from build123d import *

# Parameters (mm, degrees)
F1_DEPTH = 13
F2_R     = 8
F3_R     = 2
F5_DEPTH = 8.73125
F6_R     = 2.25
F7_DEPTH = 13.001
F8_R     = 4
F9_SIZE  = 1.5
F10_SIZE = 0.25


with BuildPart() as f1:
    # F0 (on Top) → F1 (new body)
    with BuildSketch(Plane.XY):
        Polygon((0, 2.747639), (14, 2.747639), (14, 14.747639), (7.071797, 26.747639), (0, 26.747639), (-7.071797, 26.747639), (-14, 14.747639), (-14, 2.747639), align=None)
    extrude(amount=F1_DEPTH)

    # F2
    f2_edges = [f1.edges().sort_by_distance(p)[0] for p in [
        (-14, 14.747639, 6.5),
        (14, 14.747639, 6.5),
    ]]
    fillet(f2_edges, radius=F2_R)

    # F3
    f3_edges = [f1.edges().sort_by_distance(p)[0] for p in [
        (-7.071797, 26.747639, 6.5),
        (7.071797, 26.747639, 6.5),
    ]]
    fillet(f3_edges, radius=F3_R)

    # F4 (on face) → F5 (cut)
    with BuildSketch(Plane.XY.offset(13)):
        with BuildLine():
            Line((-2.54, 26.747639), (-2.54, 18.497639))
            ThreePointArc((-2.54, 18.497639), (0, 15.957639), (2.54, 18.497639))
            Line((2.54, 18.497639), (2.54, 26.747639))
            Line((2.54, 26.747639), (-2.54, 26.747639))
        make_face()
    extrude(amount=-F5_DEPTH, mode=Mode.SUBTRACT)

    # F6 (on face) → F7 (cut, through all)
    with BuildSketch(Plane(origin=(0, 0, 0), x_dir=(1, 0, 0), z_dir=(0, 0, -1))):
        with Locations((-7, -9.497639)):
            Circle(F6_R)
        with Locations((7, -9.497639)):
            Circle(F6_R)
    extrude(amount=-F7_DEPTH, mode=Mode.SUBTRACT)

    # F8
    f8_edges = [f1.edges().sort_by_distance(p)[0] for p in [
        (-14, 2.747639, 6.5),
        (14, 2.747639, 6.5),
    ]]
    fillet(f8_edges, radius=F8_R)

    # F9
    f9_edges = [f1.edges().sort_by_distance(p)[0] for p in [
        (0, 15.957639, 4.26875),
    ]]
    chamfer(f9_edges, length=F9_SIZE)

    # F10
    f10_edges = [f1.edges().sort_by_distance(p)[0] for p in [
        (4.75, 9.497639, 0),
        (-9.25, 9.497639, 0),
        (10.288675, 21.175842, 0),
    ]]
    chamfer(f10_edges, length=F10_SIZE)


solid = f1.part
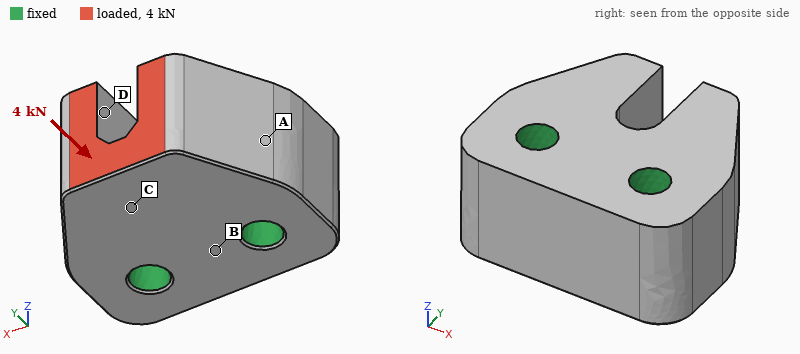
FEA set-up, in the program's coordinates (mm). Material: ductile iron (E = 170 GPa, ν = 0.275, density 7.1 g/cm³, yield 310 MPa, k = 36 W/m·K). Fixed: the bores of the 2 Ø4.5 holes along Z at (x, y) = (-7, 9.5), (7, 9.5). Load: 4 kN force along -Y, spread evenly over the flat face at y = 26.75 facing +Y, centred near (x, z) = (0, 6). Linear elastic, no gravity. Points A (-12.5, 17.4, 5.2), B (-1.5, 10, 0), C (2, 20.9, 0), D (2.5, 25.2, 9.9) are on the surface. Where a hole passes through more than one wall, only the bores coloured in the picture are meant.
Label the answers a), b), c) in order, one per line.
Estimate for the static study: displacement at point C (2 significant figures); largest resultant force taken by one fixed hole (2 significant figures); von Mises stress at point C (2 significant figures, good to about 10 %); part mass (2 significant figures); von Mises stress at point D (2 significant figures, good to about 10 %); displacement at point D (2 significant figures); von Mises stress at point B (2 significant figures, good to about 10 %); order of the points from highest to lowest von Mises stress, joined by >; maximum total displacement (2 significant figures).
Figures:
a) 1.9 µm
b) 2.1 kN
c) 32 MPa
d) 48 g
e) 42 MPa
f) 2.8 µm
g) 10 MPa
h) D > C > B > A
i) 3.5 µm
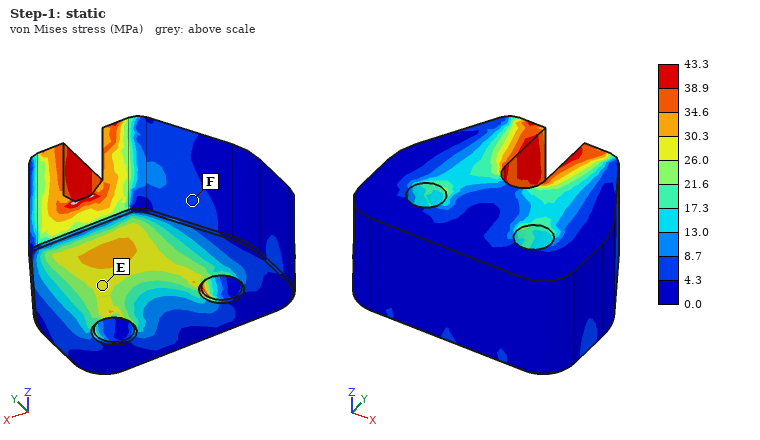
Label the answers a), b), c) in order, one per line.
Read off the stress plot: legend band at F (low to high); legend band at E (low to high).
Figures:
a) 4.3 to 8.7 MPa
b) 26.0 to 30.3 MPa
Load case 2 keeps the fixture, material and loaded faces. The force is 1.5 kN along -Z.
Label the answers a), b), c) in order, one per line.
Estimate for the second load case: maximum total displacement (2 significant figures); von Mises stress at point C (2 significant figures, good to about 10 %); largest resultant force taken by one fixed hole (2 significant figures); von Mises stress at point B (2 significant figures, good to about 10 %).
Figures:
a) 7.2 µm
b) 25 MPa
c) 750 N
d) 16 MPa
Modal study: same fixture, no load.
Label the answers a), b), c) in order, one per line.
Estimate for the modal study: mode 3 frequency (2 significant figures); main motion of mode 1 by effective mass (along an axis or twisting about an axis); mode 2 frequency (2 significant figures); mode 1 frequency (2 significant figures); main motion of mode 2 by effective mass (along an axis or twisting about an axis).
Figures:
a) 47 kHz
b) along Z
c) 39 kHz
d) 32 kHz
e) along X
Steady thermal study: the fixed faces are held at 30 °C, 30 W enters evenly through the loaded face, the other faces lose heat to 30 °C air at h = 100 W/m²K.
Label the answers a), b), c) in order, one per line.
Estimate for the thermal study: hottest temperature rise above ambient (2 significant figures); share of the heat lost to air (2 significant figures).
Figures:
a) 66 K
b) 11 %
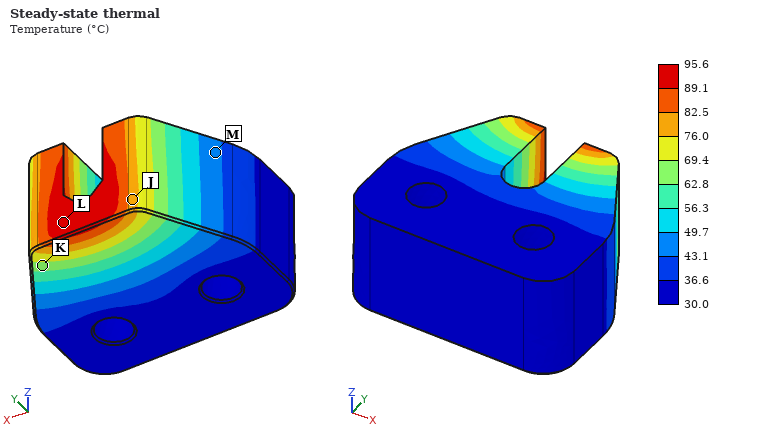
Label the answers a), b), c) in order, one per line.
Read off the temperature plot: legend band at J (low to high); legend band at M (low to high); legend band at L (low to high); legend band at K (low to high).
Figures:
a) 76.0 to 82.5 °C
b) 43.1 to 49.7 °C
c) 89.1 to 95.6 °C
d) 62.8 to 69.4 °C
